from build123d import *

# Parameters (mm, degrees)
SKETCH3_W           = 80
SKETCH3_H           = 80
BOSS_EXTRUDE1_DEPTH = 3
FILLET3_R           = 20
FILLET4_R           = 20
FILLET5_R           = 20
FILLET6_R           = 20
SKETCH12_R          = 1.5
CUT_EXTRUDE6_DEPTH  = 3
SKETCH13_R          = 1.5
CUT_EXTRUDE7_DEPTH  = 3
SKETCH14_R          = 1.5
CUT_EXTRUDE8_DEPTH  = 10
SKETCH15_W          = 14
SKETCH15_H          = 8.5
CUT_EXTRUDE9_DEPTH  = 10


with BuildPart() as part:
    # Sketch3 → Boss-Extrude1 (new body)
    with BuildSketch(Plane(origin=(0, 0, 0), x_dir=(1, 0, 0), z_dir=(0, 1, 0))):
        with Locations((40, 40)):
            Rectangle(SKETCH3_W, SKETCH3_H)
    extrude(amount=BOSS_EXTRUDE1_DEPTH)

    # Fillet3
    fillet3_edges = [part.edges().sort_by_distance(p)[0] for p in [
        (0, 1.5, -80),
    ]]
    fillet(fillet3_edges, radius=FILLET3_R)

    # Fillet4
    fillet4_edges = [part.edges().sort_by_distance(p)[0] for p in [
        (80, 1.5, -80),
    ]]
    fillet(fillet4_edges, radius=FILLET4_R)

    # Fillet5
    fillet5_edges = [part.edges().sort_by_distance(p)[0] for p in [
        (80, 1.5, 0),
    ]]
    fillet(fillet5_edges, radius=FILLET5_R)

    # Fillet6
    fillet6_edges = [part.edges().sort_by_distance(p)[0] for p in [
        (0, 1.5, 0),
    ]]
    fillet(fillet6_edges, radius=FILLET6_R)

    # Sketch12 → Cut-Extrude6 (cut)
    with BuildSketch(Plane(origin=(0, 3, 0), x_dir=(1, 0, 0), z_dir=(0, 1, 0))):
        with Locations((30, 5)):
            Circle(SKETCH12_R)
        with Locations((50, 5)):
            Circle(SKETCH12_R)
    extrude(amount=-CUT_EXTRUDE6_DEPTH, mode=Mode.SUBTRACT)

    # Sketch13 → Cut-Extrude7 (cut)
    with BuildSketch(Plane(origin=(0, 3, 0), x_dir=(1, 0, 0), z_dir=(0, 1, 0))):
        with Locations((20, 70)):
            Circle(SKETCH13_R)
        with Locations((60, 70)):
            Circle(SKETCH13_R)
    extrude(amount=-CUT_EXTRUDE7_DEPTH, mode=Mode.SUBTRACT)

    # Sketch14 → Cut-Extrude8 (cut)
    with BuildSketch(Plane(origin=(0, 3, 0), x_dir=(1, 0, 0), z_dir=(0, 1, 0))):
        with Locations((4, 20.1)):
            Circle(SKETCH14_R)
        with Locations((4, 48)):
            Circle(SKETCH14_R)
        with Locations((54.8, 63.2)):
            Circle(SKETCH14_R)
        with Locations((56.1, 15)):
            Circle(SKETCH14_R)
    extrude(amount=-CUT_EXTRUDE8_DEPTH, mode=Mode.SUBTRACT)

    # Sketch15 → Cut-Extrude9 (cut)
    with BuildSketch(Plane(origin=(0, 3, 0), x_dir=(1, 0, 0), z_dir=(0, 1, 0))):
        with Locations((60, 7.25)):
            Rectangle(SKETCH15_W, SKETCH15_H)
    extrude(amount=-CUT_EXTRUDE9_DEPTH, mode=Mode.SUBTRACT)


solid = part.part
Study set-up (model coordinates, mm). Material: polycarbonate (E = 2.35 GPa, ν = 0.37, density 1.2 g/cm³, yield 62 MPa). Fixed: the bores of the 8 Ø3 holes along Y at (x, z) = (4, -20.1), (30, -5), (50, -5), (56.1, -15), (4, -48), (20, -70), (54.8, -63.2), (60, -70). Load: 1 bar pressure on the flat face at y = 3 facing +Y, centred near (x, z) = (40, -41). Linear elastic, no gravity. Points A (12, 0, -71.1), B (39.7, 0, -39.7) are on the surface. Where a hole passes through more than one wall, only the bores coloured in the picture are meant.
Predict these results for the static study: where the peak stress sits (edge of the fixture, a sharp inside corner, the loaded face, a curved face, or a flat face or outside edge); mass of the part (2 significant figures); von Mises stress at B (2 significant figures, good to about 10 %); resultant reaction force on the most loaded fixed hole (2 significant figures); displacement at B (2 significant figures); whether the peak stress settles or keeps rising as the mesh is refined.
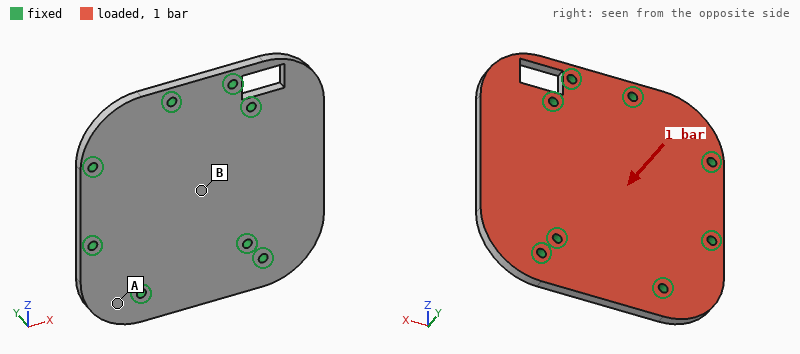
edge of the fixture
21 g
5.8 MPa
140 N
0.40 mm
keeps rising
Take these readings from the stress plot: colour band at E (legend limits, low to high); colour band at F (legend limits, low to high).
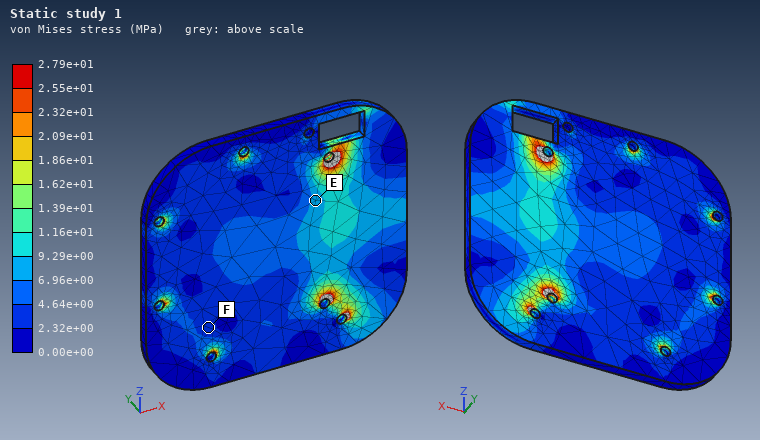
6.96e+00 to 9.29e+00 MPa
2.32e+00 to 4.64e+00 MPa
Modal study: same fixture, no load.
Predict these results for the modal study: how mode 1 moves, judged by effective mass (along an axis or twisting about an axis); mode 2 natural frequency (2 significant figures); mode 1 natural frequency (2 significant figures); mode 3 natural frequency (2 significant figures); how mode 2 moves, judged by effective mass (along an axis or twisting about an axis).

along Y
1500 Hz
960 Hz
1700 Hz
along Y
